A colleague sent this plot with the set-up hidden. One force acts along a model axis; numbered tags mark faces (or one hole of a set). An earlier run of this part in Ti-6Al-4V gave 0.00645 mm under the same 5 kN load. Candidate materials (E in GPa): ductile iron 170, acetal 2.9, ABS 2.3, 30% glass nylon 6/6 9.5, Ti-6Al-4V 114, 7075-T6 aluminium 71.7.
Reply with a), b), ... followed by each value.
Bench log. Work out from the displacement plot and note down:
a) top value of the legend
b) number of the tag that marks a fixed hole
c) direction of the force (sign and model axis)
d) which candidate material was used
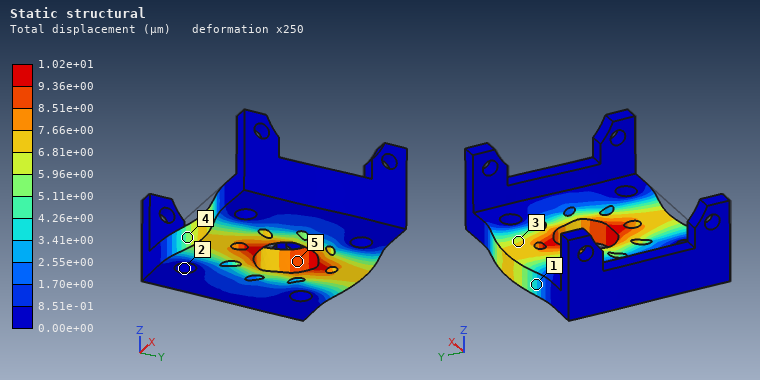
a) 1.02e+01 µm
b) 2
c) +Y
d) 7075-T6 aluminium
